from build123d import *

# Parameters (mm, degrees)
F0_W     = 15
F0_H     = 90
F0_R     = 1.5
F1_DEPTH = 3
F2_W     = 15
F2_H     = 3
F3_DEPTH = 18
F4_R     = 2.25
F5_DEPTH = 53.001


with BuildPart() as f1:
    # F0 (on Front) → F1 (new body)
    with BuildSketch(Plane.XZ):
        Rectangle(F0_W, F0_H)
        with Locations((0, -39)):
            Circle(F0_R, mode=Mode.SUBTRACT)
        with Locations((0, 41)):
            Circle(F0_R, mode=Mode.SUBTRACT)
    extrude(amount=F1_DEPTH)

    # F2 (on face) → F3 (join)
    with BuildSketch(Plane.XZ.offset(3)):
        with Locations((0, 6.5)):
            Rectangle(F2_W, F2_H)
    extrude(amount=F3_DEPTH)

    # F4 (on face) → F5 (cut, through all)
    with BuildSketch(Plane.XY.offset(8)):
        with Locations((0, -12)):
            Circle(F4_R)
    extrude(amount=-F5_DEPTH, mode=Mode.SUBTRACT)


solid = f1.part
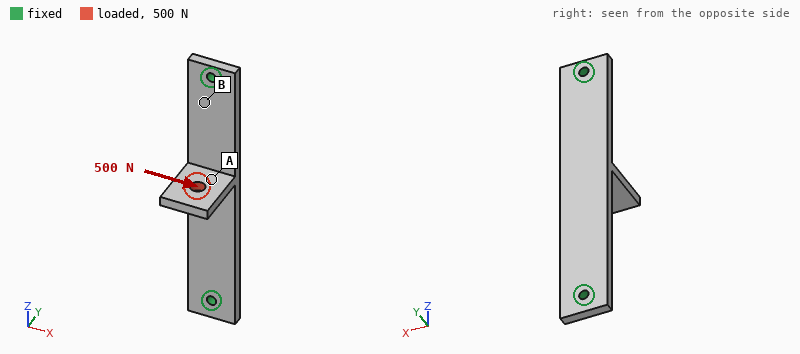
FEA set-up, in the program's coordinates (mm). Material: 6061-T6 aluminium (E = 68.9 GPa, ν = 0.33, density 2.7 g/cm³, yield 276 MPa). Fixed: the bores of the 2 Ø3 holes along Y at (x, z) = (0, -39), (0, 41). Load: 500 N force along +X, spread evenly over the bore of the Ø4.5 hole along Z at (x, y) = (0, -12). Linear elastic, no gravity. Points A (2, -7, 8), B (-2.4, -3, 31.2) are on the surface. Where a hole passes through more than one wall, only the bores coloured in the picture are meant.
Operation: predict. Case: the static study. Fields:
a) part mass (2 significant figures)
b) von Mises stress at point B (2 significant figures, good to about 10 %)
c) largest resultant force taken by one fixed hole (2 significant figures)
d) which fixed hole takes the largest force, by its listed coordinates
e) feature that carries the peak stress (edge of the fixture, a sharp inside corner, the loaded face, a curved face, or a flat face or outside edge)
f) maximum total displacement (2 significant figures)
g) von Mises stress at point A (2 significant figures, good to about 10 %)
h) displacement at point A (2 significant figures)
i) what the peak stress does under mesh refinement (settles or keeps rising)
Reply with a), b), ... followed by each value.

a) 13 g
b) 140 MPa
c) 290 N
d) (0, 41)
e) edge of the fixture
f) 0.70 mm
g) 31 MPa
h) 0.23 mm
i) keeps rising
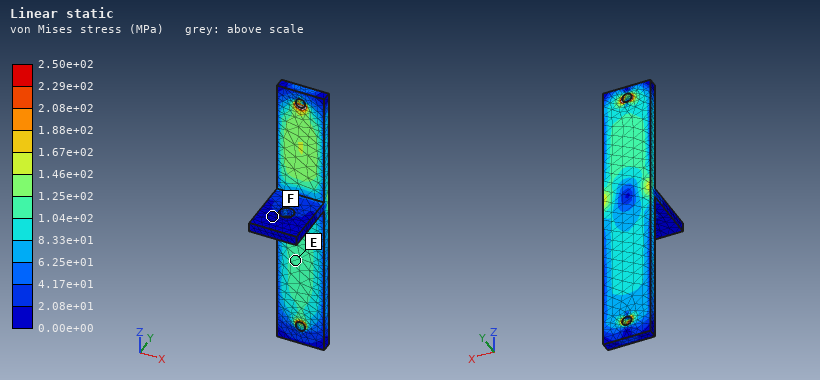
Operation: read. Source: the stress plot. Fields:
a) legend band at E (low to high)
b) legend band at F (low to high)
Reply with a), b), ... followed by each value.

a) 1.04e+02 to 1.25e+02 MPa
b) 0.00e+00 to 2.08e+01 MPa
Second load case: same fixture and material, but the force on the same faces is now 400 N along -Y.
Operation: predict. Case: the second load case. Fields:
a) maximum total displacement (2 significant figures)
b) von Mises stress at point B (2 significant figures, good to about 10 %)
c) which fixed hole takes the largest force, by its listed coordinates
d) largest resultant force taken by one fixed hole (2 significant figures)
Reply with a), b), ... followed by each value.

a) 0.43 mm
b) 81 MPa
c) (0, 41)
d) 240 N
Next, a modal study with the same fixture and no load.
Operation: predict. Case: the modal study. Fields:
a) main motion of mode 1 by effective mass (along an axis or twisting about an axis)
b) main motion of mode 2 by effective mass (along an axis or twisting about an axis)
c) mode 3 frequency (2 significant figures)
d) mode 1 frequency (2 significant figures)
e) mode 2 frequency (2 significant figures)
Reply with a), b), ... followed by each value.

a) along Y
b) along X
c) 4400 Hz
d) 2000 Hz
e) 3200 Hz
